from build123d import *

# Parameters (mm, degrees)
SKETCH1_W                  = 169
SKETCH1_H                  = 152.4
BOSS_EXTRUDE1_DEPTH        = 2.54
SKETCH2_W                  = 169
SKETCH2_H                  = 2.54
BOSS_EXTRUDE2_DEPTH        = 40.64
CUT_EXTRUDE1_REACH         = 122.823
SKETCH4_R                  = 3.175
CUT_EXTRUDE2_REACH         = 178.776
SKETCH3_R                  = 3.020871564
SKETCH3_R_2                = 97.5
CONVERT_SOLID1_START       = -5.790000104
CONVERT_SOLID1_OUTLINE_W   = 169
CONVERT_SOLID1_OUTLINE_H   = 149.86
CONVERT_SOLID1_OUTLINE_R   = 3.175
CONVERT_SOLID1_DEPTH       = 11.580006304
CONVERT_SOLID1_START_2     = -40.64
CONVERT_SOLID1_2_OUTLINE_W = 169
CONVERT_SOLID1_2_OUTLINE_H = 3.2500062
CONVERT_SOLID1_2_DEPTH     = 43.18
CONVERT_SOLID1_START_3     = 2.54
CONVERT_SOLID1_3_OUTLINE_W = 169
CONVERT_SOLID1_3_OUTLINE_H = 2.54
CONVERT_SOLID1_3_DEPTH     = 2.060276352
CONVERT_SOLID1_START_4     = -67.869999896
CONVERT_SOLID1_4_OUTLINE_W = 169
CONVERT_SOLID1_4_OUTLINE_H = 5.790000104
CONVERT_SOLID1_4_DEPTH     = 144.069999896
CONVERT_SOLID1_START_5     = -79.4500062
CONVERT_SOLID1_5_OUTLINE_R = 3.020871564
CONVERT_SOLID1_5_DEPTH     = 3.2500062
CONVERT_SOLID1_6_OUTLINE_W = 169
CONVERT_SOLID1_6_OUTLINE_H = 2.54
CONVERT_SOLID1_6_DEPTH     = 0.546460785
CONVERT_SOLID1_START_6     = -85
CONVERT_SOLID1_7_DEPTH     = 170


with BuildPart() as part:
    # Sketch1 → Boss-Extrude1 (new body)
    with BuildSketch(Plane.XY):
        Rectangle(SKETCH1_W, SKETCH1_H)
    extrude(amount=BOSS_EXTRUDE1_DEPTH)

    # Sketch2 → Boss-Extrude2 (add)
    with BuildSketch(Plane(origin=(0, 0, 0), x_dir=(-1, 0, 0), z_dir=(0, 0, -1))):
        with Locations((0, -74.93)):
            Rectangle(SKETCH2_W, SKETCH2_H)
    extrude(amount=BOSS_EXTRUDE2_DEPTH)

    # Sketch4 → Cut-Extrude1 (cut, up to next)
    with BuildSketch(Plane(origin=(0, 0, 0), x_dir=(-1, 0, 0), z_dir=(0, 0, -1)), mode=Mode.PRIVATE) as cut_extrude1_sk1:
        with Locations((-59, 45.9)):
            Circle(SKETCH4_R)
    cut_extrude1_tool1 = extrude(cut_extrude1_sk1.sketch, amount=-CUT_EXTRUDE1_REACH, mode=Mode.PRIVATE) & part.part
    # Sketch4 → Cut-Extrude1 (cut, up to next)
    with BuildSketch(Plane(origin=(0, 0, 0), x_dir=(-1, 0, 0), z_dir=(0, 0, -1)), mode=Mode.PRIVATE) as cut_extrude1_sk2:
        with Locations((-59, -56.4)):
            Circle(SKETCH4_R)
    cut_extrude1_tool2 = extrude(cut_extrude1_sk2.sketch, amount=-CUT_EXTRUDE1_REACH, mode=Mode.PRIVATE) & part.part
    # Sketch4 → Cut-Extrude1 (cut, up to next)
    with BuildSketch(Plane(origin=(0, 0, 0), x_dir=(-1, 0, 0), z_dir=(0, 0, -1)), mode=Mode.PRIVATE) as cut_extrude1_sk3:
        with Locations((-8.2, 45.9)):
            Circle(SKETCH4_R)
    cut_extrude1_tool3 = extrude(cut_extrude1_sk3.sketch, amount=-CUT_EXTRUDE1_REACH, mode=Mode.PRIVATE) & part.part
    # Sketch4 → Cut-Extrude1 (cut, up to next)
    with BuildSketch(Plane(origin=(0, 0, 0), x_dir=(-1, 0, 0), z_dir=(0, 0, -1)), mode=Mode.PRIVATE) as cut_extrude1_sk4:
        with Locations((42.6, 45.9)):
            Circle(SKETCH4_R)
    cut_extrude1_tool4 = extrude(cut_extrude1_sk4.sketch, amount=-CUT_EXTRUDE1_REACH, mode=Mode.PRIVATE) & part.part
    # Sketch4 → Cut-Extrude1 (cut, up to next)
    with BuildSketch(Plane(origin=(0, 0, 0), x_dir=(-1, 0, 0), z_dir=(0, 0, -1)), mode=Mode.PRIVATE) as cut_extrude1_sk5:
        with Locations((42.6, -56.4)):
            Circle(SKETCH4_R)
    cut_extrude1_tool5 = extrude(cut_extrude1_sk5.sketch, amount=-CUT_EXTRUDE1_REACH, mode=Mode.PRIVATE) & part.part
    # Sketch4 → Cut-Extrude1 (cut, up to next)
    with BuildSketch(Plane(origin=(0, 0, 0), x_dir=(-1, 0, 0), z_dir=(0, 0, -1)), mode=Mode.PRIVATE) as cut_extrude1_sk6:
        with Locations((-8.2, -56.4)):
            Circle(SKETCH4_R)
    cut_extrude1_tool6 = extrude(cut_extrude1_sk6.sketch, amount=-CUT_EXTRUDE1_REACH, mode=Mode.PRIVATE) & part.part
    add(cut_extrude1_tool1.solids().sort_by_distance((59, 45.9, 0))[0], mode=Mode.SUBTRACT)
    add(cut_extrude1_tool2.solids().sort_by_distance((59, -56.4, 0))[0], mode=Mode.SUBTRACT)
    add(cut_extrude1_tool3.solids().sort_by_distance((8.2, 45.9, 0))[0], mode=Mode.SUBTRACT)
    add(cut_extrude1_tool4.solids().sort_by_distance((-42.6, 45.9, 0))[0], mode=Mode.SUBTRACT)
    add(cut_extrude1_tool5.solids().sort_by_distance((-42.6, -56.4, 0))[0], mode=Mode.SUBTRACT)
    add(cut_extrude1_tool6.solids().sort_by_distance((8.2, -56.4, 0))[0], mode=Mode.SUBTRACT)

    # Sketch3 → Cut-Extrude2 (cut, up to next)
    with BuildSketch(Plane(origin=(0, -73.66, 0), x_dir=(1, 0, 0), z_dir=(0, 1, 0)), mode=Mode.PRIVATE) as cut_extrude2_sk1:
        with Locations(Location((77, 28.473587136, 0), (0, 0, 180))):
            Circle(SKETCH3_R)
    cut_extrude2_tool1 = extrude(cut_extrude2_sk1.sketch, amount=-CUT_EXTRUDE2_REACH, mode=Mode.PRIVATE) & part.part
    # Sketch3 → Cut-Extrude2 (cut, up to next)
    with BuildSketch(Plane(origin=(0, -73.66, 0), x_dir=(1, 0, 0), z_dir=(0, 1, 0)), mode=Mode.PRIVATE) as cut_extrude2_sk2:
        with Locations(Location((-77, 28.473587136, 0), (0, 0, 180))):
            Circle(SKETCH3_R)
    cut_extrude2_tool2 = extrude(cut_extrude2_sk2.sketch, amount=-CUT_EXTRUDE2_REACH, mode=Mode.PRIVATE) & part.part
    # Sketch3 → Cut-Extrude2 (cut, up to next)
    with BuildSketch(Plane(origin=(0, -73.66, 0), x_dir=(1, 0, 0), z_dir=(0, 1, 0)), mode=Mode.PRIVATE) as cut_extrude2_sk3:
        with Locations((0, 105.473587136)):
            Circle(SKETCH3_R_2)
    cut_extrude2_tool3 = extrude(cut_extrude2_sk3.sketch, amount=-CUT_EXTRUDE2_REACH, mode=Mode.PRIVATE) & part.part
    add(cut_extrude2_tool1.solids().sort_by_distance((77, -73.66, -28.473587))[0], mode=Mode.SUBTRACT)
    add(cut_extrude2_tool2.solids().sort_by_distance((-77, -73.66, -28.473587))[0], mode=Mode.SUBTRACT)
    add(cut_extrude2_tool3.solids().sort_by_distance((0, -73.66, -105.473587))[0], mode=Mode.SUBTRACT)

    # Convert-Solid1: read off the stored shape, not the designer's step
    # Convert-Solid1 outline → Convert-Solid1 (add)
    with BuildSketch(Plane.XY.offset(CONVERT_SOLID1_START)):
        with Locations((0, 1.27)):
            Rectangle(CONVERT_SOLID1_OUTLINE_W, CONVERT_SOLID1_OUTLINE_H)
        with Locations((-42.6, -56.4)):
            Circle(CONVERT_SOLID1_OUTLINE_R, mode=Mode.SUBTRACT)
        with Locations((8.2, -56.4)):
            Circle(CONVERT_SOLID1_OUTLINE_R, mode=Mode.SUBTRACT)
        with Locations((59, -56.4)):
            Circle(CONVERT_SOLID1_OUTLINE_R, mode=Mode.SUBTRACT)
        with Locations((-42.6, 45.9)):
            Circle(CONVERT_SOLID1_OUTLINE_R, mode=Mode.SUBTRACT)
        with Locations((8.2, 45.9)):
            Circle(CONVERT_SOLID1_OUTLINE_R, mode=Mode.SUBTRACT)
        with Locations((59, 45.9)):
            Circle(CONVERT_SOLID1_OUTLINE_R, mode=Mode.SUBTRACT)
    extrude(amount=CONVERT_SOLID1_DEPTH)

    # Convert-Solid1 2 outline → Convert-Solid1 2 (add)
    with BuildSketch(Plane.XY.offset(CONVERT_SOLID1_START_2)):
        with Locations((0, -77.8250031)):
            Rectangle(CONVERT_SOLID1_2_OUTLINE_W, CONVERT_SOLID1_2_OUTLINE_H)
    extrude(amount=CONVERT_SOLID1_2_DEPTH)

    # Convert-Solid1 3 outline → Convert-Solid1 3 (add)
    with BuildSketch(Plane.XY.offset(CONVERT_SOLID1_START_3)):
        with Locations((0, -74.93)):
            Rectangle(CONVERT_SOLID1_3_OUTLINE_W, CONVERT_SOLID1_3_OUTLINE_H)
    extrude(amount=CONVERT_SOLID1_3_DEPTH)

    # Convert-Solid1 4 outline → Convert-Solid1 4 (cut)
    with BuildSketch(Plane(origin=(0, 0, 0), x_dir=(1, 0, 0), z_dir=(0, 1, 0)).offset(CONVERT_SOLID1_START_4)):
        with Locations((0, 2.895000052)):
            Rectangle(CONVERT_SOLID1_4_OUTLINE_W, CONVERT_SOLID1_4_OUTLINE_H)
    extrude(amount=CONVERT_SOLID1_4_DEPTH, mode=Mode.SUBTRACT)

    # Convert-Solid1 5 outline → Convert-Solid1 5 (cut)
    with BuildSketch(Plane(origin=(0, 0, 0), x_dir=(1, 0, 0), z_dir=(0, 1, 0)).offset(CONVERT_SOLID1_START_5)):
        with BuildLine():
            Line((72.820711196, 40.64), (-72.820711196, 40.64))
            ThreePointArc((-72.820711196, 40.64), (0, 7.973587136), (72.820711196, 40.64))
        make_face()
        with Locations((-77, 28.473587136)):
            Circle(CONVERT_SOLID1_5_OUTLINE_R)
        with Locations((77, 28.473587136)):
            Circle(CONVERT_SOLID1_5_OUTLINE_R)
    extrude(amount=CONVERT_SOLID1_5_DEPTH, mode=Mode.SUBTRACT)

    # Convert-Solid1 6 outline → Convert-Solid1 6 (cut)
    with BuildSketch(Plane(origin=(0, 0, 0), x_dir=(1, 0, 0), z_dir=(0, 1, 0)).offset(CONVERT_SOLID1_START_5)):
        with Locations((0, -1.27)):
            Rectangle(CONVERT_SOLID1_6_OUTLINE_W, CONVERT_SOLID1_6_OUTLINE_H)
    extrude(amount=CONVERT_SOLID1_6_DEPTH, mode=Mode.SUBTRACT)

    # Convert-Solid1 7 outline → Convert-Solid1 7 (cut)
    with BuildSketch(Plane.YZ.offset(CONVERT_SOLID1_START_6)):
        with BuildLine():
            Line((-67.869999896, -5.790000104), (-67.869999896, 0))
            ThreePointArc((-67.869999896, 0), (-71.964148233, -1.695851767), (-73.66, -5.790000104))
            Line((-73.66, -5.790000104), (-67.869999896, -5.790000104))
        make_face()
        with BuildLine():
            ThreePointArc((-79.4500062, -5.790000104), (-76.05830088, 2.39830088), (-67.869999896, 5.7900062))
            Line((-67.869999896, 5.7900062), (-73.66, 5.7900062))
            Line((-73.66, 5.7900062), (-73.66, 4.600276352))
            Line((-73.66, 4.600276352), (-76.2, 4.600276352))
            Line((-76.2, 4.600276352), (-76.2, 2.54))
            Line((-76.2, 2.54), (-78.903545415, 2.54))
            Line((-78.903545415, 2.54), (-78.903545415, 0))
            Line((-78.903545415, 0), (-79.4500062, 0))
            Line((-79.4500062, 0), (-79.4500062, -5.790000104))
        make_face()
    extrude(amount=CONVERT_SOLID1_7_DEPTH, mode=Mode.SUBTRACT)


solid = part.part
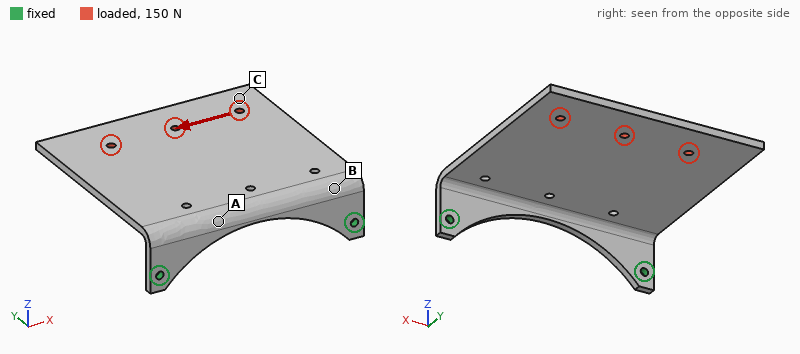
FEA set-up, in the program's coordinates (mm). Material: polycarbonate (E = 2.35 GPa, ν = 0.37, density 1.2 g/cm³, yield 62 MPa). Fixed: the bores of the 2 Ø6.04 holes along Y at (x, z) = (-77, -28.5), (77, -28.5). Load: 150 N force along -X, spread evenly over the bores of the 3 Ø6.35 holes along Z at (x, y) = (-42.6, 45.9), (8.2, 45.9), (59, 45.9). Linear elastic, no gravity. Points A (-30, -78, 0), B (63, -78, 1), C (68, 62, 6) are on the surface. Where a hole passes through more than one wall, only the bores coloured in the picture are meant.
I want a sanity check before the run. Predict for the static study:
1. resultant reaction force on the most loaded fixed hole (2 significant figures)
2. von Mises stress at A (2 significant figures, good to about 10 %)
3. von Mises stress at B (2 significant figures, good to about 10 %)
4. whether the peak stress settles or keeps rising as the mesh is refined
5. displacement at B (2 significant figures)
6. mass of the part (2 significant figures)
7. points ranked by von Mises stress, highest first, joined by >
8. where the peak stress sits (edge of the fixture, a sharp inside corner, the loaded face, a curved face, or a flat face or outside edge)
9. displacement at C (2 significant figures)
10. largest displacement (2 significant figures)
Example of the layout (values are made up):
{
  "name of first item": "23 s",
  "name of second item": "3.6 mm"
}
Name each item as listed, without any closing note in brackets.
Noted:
{
  "resultant reaction force on the most loaded fixed hole": "140 N",
  "von Mises stress at A": "2.6 MPa",
  "von Mises stress at B": "3.9 MPa",
  "whether the peak stress settles or keeps rising as the mesh is refined": "keeps rising",
  "displacement at B": "0.54 mm",
  "mass of the part": "200 g",
  "points ranked by von Mises stress, highest first, joined by >": "B > A > C",
  "where the peak stress sits": "edge of the fixture",
  "displacement at C": "1.8 mm",
  "largest displacement": "2.2 mm"
}
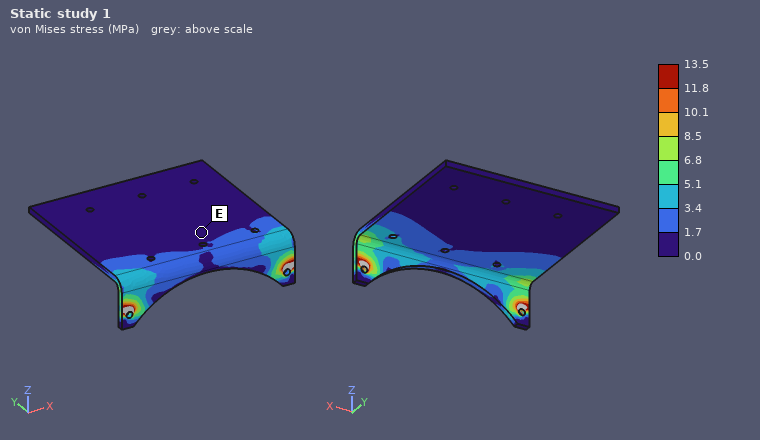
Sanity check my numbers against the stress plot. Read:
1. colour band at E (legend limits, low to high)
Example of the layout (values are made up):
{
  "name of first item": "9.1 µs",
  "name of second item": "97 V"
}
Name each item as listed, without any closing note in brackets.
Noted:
{
  "colour band at E": "0.0 to 1.7 MPa"
}
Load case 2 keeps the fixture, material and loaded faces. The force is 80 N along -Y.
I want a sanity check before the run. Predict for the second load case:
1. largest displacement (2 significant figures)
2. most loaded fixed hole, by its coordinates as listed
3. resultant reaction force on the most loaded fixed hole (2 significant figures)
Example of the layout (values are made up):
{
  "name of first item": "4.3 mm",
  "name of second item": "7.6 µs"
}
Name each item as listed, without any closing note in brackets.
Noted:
{
  "largest displacement": "2.6 mm",
  "most loaded fixed hole, by its coordinates as listed": "(77, -28.5)",
  "resultant reaction force on the most loaded fixed hole": "44 N"
}
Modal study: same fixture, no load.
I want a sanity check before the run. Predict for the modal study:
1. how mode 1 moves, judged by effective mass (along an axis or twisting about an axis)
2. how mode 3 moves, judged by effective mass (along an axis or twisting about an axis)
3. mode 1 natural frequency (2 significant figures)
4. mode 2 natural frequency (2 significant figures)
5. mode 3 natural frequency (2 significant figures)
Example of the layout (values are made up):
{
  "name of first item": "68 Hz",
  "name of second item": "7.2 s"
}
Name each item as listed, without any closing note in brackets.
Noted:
{
  "how mode 1 moves, judged by effective mass": "along Z",
  "how mode 3 moves, judged by effective mass": "along X",
  "mode 1 natural frequency": "32 Hz",
  "mode 2 natural frequency": "100 Hz",
  "mode 3 natural frequency": "180 Hz"
}
